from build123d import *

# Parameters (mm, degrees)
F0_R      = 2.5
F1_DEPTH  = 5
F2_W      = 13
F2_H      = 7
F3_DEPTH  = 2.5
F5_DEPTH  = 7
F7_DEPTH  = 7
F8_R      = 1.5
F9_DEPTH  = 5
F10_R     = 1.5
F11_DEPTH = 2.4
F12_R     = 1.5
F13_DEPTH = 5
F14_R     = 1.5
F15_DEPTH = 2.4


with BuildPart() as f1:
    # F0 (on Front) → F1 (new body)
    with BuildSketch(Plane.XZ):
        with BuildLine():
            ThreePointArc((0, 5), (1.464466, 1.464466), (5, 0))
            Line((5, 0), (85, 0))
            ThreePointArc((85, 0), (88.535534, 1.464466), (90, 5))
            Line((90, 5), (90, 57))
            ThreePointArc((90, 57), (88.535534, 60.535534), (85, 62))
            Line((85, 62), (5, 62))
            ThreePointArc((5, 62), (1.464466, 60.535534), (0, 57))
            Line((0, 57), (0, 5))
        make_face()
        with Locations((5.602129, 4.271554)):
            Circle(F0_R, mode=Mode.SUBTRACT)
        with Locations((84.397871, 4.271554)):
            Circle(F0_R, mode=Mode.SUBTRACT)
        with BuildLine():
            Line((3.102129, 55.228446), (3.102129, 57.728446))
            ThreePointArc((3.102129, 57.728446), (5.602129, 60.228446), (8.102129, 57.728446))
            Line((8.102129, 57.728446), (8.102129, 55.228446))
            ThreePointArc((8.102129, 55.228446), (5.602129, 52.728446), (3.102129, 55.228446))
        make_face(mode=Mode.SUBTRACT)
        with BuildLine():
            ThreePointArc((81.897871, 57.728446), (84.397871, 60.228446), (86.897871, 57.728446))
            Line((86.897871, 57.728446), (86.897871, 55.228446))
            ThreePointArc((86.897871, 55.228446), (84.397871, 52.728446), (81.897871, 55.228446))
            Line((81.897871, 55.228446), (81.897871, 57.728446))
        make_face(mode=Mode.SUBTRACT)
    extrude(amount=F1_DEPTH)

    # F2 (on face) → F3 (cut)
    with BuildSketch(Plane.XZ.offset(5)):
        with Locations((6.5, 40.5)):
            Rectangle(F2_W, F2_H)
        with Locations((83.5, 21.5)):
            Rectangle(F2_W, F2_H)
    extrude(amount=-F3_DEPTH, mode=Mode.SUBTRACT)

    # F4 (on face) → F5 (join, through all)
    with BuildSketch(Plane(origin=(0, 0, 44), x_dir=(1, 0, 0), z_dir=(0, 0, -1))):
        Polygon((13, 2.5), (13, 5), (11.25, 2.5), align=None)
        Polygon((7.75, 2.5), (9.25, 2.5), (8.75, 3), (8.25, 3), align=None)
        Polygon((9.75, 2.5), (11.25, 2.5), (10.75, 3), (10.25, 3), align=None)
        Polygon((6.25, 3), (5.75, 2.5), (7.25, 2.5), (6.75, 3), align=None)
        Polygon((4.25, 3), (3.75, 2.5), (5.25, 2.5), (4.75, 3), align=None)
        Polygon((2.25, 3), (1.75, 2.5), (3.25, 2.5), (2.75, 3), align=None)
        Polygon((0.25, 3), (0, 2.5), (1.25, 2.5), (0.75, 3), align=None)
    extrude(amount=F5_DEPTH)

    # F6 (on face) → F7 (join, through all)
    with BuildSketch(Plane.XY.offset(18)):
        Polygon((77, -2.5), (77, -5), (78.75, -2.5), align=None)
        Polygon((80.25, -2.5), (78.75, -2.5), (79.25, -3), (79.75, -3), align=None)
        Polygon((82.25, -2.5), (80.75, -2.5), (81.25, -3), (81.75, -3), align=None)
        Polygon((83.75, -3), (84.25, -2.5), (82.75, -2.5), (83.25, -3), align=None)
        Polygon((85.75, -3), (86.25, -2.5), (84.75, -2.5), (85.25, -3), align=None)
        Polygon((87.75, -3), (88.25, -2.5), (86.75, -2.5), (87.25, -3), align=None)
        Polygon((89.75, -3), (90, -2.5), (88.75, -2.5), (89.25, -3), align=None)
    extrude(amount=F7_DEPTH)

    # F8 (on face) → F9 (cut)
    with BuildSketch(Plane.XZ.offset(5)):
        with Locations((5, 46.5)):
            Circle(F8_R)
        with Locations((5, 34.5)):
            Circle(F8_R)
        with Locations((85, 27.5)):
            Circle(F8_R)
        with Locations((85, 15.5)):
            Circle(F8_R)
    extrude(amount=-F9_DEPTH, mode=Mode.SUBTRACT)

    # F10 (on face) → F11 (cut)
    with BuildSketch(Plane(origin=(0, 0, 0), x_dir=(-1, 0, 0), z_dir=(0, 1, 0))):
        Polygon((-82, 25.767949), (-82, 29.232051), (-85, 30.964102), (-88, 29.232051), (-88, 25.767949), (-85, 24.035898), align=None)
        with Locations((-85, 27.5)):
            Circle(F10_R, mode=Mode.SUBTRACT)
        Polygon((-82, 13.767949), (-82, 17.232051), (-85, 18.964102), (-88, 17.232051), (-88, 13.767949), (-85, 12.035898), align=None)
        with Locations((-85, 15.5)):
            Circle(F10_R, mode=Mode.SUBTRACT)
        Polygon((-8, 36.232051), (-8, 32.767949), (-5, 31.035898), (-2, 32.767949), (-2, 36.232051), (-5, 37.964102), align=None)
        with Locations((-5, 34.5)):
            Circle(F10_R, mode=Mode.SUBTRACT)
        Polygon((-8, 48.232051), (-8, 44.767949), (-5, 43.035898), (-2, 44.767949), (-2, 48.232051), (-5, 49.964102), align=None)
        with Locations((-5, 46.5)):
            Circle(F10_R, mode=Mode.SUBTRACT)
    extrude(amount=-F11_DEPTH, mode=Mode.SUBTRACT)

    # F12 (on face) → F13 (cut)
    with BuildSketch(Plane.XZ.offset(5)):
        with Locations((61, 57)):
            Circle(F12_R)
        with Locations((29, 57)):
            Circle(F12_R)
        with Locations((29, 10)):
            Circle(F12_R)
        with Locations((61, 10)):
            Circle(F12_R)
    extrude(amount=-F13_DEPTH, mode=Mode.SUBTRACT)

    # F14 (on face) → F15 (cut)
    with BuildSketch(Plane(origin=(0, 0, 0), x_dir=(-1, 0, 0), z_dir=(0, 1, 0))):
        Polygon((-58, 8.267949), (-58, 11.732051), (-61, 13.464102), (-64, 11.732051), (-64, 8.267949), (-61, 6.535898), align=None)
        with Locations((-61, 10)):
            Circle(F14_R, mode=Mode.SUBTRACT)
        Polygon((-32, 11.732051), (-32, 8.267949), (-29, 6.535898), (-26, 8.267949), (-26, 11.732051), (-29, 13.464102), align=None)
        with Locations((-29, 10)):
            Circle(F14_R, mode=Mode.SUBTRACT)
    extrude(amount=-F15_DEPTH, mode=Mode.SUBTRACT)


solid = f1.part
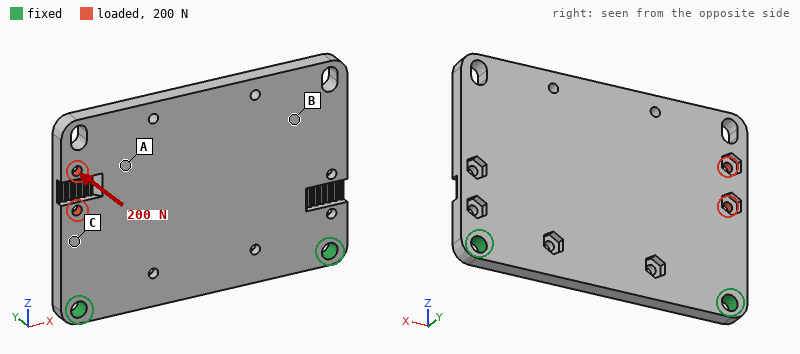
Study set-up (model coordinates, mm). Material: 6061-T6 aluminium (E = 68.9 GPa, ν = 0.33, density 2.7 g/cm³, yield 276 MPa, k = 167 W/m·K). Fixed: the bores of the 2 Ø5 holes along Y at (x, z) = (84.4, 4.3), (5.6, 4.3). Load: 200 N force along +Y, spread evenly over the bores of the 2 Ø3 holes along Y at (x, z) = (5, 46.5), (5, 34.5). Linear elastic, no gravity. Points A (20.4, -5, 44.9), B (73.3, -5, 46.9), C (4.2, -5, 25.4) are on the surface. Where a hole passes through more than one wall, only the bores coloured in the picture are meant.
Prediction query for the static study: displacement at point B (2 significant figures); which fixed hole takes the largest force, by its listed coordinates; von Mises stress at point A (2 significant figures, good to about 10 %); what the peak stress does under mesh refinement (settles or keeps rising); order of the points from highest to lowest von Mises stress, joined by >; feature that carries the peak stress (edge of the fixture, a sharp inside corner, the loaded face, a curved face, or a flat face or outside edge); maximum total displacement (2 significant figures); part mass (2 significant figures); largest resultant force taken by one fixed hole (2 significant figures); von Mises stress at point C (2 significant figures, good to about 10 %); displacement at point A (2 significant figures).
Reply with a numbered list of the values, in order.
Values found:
1. 0.086 mm
2. (5.6, 4.3)
3. 11 MPa
4. keeps rising
5. C > A > B
6. edge of the fixture
7. 0.25 mm
8. 71 g
9. 210 N
10. 23 MPa
11. 0.15 mm
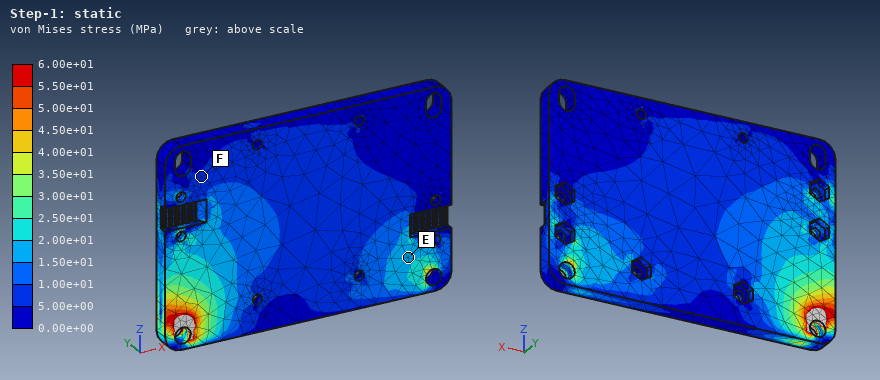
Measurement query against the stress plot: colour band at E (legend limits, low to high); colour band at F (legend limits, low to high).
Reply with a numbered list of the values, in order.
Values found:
1. 1.50e+01 to 2.00e+01 MPa
2. 5.00e+00 to 1.00e+01 MPa
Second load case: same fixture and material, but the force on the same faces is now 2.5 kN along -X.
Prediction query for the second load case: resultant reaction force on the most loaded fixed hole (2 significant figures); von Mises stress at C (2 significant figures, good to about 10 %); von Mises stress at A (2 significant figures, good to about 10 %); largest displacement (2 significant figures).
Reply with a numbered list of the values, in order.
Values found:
1. 1.7 kN
2. 24 MPa
3. 27 MPa
4. 51 µm
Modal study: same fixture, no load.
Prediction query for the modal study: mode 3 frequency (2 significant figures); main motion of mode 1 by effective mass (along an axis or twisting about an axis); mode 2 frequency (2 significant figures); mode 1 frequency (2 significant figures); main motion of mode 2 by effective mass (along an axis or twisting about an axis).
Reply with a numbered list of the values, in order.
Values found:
1. 3800 Hz
2. along Y
3. 2200 Hz
4. 850 Hz
5. twisting about Z
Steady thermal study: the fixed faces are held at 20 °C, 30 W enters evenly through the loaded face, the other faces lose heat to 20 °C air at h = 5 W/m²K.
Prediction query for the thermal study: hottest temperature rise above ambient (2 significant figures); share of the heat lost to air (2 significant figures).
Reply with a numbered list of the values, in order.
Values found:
1. 52 K
2. 3.8 %
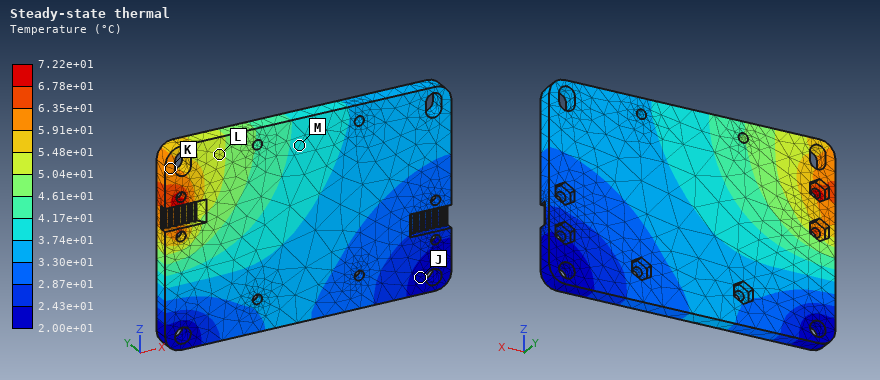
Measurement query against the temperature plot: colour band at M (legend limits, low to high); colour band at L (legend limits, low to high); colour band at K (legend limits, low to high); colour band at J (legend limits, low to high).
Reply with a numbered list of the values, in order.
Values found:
1. 3.74e+01 to 4.17e+01 °C
2. 5.04e+01 to 5.48e+01 °C
3. 5.91e+01 to 6.35e+01 °C
4. 2.00e+01 to 2.43e+01 °C
